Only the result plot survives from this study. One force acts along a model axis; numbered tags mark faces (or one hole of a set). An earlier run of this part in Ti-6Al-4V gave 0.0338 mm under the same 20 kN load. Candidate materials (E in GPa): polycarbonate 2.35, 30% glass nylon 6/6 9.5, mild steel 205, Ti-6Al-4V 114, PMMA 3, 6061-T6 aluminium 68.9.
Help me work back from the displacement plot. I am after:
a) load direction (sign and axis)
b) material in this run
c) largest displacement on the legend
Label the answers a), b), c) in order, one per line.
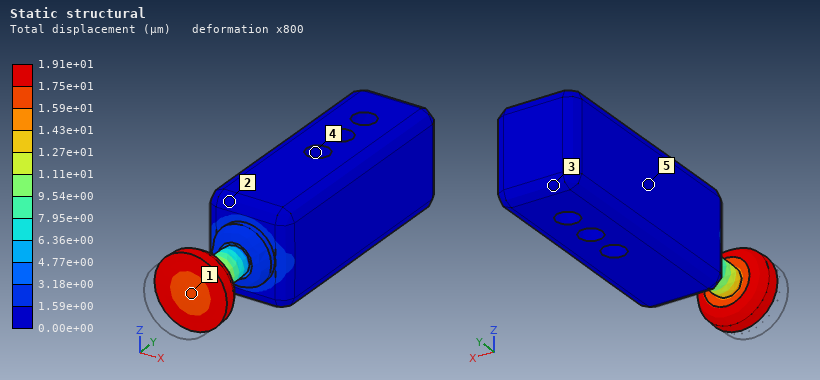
a) +Y
b) mild steel
c) 1.91e+01 µm
